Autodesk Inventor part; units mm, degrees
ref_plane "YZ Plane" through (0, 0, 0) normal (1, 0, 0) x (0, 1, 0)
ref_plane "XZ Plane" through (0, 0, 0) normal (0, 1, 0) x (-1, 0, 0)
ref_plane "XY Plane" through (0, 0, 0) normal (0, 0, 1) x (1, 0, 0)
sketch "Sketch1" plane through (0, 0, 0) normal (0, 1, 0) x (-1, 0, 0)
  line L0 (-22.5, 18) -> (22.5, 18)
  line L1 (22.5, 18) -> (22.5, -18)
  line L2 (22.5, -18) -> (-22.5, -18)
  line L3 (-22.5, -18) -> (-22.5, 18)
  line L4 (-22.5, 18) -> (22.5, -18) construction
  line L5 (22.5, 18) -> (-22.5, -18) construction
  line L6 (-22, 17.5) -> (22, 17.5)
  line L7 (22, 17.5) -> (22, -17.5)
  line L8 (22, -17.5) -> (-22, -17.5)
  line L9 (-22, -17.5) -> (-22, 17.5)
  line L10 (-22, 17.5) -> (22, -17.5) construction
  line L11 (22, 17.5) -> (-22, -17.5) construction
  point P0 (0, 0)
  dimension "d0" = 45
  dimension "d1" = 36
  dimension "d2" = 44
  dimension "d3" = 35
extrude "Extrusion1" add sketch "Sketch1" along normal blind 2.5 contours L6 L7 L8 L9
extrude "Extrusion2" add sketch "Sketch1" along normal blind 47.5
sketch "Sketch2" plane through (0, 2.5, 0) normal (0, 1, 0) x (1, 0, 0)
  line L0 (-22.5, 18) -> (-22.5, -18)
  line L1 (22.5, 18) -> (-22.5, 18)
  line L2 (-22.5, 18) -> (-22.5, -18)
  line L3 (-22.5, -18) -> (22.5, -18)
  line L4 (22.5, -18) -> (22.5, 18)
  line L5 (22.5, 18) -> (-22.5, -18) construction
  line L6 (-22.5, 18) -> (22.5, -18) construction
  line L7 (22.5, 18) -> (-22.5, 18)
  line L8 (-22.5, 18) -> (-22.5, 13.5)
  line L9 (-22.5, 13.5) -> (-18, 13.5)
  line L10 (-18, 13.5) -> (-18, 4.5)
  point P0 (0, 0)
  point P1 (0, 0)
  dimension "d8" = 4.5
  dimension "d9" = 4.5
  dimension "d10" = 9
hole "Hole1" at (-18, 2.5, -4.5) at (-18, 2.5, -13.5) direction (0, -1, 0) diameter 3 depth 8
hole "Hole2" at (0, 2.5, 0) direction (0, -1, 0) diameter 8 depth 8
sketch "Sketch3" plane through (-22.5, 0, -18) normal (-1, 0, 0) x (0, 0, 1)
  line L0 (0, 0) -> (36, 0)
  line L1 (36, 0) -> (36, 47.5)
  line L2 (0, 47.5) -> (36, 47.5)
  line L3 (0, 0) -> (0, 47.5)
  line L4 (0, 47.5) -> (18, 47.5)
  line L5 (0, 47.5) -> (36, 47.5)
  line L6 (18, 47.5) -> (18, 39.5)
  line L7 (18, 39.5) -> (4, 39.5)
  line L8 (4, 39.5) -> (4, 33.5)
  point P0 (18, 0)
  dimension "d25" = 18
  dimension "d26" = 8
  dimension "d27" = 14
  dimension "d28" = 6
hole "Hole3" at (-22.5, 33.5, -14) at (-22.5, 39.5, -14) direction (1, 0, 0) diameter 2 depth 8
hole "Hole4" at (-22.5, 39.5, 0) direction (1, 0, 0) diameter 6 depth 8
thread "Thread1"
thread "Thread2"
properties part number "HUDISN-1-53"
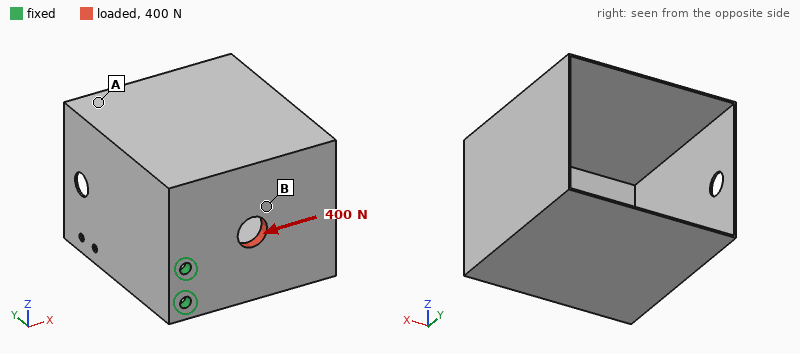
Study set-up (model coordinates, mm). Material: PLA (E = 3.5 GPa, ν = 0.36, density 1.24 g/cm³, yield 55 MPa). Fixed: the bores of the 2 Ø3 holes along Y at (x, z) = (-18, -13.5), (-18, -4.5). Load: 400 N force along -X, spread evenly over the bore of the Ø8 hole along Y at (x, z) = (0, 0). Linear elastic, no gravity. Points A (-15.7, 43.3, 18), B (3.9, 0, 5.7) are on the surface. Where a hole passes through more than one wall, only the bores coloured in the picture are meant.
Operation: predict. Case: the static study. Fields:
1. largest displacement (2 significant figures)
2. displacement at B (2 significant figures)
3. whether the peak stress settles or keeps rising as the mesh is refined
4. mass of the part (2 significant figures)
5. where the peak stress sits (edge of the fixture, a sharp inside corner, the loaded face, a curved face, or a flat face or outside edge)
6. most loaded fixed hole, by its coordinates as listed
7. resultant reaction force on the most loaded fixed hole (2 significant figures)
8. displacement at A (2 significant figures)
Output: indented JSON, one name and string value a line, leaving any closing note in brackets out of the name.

{
  "largest displacement": "0.41 mm",
  "displacement at B": "0.22 mm",
  "whether the peak stress settles or keeps rising as the mesh is refined": "keeps rising",
  "mass of the part": "9.3 g",
  "where the peak stress sits": "edge of the fixture",
  "most loaded fixed hole, by its coordinates as listed": "(-18, -4.5)",
  "resultant reaction force on the most loaded fixed hole": "510 N",
  "displacement at A": "0.26 mm"
}
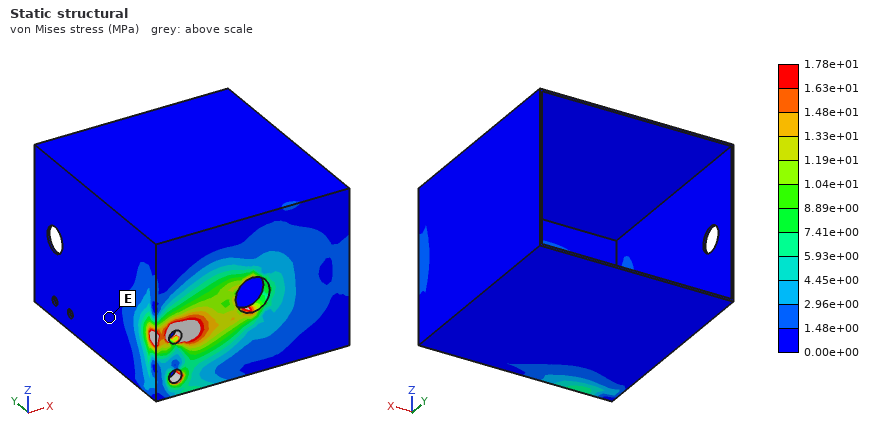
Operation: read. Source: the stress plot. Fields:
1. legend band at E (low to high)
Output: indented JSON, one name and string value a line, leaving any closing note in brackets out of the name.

{
  "legend band at E": "0.00e+00 to 1.48e+00 MPa"
}
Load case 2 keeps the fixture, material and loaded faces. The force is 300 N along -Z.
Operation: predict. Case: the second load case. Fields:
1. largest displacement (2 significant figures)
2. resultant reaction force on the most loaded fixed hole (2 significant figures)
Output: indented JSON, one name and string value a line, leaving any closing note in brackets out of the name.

{
  "largest displacement": "0.65 mm",
  "resultant reaction force on the most loaded fixed hole": "480 N"
}
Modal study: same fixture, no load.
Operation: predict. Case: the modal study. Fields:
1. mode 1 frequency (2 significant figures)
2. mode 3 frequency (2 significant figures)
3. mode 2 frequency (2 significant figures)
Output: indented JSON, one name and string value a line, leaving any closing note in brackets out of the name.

{
  "mode 1 frequency": "230 Hz",
  "mode 3 frequency": "360 Hz",
  "mode 2 frequency": "290 Hz"
}
